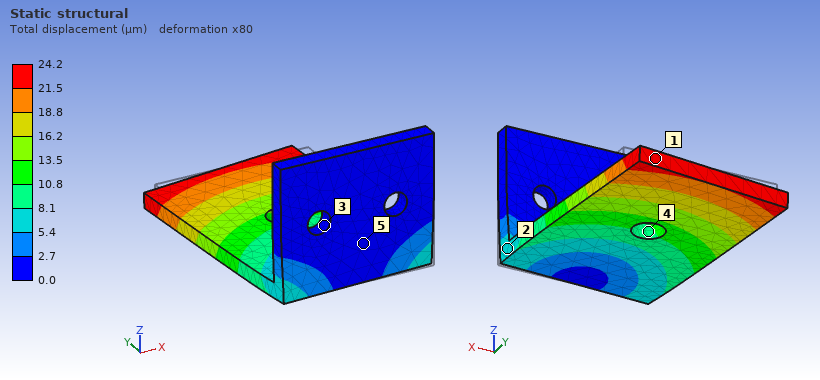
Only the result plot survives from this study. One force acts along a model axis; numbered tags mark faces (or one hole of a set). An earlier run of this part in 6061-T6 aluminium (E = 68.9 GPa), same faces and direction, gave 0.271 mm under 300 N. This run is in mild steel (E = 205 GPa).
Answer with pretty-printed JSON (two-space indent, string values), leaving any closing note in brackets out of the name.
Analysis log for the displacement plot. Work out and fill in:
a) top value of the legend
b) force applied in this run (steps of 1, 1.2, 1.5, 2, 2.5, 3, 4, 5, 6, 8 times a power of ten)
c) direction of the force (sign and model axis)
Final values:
{
  "top value of the legend": "24.2 µm",
  "force applied in this run": "80 N",
  "direction of the force": "-X"
}
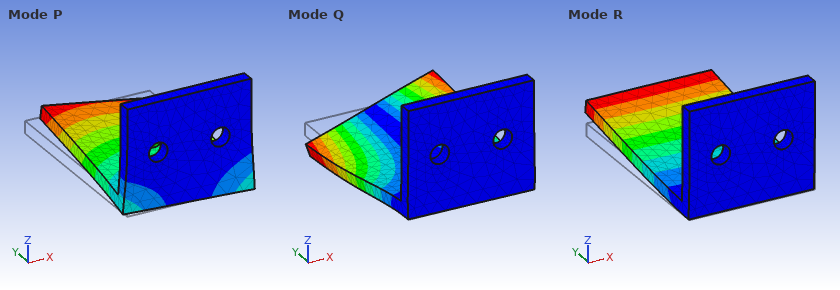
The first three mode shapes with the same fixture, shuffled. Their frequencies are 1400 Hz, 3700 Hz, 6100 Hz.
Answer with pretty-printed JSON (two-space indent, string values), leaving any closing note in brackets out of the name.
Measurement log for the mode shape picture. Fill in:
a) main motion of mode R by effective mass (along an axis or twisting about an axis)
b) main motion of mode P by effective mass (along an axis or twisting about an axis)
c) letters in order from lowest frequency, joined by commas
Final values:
{
  "main motion of mode R by effective mass": "along Z",
  "main motion of mode P by effective mass": "along X",
  "letters in order from lowest frequency, joined by commas": "R, P, Q"
}
